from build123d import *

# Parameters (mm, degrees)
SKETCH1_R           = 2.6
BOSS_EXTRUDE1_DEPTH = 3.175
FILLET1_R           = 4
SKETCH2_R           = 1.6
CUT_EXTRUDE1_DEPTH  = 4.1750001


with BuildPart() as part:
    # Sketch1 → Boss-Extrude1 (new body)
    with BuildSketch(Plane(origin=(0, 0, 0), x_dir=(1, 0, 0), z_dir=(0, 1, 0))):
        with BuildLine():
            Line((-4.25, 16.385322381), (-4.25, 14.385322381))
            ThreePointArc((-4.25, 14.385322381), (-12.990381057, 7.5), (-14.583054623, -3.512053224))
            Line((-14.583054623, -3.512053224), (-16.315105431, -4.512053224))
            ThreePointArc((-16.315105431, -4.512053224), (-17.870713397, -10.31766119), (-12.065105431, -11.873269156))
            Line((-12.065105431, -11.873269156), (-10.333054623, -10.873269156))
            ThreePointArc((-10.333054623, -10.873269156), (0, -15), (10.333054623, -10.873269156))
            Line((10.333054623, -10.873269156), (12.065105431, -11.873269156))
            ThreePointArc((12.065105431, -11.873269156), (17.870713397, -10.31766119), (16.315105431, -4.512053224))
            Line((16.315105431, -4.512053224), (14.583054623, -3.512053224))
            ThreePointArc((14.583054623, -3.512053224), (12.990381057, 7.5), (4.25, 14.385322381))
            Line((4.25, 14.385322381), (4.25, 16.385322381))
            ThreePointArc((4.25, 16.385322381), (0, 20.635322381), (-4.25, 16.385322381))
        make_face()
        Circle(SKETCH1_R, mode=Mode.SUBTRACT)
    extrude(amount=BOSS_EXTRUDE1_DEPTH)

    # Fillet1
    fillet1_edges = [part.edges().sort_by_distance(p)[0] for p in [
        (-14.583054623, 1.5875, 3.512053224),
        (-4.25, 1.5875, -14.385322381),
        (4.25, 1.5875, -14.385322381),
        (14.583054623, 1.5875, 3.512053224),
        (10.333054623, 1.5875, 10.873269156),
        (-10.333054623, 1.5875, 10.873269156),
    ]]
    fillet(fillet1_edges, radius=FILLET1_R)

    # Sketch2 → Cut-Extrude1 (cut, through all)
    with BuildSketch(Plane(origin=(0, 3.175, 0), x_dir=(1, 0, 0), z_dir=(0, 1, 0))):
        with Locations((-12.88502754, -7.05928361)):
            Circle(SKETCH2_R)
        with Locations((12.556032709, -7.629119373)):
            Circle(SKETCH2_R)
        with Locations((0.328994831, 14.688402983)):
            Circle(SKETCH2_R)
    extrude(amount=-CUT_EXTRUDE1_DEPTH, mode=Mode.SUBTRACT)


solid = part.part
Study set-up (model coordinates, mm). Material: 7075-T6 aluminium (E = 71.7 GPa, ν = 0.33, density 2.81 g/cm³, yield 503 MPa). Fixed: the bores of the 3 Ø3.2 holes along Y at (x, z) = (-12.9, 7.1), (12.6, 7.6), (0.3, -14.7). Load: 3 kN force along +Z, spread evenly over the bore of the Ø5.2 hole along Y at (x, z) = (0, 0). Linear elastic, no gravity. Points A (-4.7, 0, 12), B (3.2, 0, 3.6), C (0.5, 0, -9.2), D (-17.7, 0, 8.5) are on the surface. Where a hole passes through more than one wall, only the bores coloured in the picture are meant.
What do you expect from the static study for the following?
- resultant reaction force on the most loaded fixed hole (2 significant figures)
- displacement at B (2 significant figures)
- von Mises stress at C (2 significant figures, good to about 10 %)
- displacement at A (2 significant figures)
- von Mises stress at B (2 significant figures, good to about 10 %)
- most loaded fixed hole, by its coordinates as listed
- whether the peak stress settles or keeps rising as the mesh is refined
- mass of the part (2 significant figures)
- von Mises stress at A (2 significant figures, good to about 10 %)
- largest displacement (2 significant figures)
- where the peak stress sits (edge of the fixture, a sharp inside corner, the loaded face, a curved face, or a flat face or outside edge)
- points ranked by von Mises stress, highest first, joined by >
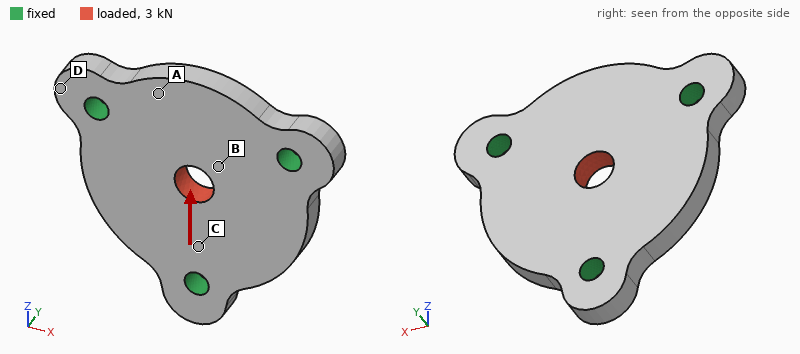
1.2 kN
8.5 µm
58 MPa
6.8 µm
40 MPa
(0.3, -14.7)
keeps rising
7.1 g
23 MPa
12 µm
edge of the fixture
C > B > A > D
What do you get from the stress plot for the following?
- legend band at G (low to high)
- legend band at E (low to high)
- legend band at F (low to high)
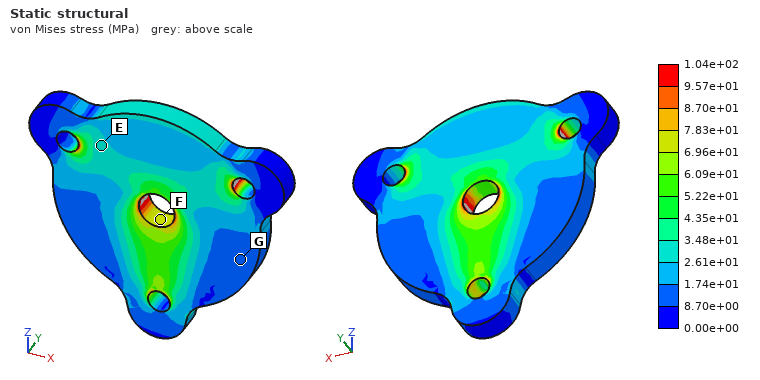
8.70e+00 to 1.74e+01 MPa
2.61e+01 to 3.48e+01 MPa
6.96e+01 to 7.83e+01 MPa
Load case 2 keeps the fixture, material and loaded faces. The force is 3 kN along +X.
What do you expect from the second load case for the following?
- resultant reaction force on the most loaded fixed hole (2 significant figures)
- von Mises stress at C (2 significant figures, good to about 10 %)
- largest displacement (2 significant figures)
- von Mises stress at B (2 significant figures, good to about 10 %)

1.2 kN
12 MPa
11 µm
49 MPa
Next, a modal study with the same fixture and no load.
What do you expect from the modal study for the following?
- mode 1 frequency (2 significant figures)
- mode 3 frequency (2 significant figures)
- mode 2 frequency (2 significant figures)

22 kHz
22 kHz
22 kHz
